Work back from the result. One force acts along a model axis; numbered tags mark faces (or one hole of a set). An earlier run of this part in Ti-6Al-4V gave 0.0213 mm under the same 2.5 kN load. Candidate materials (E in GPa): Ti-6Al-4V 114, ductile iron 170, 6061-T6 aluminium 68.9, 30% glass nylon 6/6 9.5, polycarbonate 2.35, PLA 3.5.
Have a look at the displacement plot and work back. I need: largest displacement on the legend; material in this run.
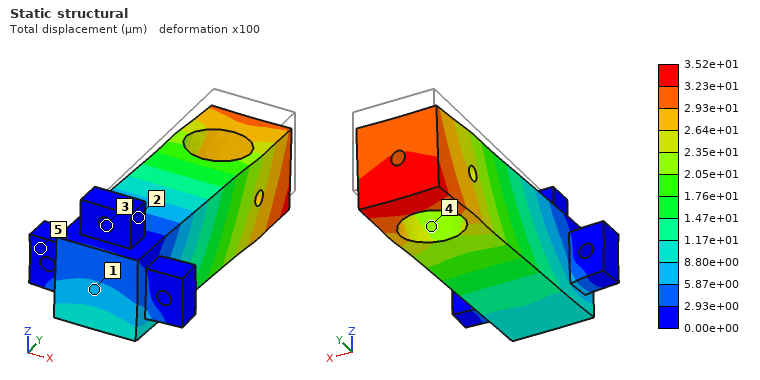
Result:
3.52e+01 µm
6061-T6 aluminium
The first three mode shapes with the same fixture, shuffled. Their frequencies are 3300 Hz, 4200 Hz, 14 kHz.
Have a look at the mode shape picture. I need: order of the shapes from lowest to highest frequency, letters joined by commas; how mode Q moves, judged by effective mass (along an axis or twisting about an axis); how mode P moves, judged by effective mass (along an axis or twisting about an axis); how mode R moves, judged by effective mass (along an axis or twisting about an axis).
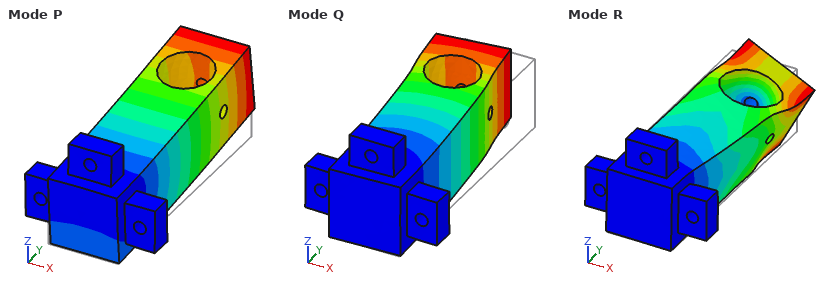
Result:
P, Q, R
along X
along Z
twisting about Y
